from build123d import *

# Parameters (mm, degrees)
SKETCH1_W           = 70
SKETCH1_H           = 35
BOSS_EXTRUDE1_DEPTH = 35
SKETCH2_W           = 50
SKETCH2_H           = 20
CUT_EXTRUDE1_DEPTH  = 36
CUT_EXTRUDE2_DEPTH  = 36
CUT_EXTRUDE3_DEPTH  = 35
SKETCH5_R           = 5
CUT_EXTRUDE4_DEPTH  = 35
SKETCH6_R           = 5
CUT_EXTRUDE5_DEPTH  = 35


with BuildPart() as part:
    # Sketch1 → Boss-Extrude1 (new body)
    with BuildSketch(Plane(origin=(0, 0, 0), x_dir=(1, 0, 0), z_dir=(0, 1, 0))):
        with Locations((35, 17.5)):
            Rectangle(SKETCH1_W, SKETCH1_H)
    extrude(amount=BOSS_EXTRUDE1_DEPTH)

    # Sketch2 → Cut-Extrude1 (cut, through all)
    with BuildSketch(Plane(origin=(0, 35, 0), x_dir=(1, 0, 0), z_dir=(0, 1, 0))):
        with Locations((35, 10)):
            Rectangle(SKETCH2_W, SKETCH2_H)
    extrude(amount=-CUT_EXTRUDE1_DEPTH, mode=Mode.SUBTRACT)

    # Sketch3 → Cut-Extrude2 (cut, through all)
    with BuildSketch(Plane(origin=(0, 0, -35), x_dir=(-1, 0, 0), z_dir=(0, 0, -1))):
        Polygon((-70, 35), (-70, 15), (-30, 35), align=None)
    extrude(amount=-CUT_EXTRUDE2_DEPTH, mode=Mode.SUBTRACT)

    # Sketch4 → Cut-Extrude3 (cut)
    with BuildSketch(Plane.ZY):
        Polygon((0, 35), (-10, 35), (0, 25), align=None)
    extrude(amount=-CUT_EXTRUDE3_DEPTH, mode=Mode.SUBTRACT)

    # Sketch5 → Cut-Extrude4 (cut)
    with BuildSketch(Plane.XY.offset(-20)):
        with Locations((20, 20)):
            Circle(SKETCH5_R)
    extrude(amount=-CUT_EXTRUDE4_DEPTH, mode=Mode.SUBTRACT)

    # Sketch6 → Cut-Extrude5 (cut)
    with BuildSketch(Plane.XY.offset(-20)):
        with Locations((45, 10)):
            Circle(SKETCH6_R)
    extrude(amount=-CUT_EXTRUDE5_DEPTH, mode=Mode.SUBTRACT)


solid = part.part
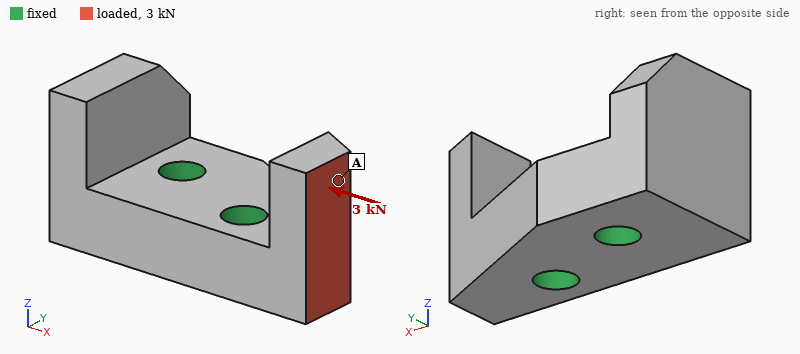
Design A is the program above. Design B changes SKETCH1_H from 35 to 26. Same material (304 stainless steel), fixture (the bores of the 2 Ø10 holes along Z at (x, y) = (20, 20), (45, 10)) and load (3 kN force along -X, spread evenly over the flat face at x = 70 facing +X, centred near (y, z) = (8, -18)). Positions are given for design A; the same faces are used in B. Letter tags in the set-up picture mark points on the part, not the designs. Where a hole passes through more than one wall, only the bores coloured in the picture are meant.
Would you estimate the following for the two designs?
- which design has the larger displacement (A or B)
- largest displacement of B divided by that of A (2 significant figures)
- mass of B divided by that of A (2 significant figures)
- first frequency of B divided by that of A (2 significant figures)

B
1.1
0.73
0.97
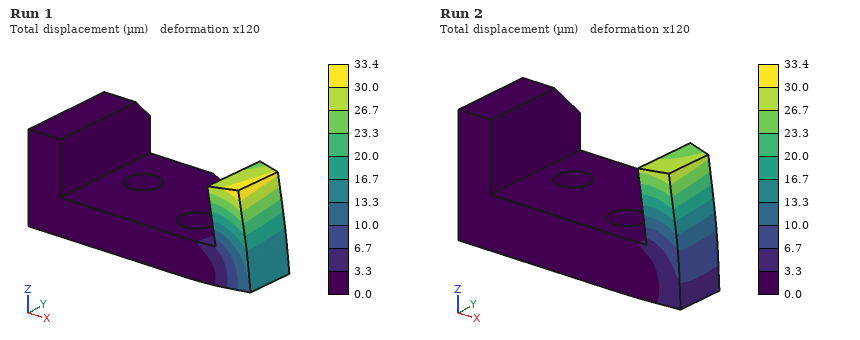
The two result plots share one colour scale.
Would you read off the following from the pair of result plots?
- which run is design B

Run 1
